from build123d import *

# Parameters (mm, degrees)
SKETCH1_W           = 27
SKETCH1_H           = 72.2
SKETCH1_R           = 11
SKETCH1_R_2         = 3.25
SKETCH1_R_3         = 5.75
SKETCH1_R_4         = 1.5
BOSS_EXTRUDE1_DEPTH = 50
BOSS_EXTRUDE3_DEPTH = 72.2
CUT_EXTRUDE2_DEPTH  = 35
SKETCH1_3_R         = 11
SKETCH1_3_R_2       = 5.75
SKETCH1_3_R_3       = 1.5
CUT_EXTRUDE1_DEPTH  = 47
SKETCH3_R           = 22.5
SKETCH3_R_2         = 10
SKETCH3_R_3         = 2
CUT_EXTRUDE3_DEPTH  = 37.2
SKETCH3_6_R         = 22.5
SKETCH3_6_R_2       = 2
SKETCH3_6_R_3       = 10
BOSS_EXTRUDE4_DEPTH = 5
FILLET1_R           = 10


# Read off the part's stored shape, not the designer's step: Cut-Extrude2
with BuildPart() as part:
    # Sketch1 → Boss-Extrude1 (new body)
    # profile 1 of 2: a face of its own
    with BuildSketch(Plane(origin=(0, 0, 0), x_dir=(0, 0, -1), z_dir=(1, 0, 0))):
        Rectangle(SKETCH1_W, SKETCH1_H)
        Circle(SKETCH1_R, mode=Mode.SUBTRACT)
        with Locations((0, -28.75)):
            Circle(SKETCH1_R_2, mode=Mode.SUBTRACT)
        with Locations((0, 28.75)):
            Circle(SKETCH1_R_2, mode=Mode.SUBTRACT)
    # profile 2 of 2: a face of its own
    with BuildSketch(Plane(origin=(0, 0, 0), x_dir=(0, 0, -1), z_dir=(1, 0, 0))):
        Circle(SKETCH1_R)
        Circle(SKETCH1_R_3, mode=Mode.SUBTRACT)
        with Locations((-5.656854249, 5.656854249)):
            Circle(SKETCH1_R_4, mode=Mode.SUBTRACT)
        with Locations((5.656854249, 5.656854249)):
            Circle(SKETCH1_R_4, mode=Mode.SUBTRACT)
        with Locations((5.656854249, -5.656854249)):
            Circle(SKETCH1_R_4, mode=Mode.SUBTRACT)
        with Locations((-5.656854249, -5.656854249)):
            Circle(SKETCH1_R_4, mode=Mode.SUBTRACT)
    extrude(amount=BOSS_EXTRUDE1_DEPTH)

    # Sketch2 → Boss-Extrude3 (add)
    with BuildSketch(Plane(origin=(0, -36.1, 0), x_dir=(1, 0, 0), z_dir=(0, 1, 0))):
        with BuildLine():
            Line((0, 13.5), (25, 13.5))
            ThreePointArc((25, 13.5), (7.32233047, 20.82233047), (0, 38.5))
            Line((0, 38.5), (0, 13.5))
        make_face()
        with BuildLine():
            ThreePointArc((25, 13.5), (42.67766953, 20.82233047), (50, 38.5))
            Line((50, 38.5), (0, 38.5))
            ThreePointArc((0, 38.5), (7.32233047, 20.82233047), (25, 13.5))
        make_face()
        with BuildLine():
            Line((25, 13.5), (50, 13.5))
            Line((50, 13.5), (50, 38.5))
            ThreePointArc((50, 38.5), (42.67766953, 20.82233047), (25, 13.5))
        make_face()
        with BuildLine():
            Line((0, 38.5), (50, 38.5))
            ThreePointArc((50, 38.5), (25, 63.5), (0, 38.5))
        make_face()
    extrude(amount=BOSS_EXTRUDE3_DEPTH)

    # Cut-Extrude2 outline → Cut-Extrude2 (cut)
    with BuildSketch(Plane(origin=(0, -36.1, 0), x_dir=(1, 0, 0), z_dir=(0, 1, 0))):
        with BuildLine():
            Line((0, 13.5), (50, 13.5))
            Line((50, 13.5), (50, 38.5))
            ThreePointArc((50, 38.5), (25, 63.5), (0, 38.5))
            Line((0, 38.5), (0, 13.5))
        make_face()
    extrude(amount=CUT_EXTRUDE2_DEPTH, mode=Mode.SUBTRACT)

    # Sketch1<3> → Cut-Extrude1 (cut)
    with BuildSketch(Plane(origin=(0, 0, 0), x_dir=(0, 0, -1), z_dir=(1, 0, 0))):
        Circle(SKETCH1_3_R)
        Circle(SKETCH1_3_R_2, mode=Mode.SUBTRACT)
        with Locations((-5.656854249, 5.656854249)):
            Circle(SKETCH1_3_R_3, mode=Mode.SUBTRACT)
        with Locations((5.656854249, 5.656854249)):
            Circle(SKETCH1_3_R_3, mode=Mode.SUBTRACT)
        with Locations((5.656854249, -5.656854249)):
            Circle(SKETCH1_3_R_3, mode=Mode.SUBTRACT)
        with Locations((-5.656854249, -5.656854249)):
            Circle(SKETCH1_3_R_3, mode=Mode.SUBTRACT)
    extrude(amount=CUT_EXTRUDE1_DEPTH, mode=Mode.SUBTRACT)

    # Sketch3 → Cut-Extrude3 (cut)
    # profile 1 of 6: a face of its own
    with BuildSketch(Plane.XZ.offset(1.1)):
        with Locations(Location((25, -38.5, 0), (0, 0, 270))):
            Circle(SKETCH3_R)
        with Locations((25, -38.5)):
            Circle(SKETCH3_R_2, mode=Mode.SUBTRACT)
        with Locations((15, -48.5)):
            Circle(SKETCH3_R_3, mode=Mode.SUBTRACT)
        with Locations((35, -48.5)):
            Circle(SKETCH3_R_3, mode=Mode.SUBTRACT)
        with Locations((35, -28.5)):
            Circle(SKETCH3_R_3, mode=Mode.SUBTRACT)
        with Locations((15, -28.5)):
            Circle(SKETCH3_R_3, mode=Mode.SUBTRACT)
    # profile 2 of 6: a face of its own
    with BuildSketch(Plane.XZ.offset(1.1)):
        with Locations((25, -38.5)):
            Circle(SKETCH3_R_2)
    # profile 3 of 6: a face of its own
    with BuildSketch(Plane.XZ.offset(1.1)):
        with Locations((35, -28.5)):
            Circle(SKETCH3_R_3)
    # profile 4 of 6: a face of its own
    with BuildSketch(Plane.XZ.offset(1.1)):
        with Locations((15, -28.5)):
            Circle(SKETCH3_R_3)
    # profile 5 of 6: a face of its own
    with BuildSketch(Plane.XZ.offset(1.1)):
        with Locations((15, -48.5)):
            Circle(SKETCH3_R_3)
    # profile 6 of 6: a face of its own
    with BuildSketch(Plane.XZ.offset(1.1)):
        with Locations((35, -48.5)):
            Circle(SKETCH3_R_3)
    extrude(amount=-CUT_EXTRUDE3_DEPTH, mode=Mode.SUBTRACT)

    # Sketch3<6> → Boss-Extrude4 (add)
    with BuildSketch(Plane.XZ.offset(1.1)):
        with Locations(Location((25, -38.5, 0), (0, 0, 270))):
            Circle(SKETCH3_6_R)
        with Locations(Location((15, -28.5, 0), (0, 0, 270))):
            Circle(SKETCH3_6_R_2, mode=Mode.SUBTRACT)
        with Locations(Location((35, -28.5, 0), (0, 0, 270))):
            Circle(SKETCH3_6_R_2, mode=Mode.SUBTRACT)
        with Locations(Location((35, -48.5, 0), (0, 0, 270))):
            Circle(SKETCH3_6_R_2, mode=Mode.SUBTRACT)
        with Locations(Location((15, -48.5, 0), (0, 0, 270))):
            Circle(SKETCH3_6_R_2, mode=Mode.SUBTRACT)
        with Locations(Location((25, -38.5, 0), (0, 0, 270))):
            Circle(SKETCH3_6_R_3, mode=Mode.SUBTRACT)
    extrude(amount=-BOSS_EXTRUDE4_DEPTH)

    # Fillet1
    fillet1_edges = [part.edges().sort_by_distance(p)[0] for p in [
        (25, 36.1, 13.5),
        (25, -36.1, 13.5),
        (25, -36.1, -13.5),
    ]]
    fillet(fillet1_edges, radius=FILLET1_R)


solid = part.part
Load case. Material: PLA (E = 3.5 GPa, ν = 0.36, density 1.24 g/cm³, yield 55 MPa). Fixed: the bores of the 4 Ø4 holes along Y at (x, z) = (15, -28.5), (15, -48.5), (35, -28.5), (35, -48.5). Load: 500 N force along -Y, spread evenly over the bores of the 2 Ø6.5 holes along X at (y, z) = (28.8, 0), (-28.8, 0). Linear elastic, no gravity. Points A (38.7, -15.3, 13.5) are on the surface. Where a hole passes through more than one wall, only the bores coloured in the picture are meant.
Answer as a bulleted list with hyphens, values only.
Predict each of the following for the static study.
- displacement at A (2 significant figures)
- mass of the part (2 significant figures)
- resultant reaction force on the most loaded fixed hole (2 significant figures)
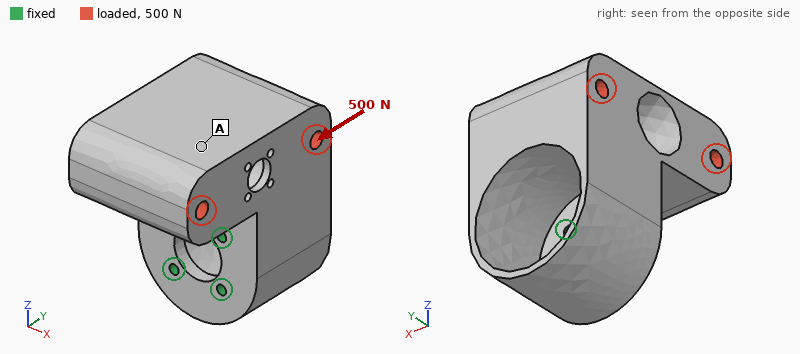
- 0.47 mm
- 130 g
- 460 N
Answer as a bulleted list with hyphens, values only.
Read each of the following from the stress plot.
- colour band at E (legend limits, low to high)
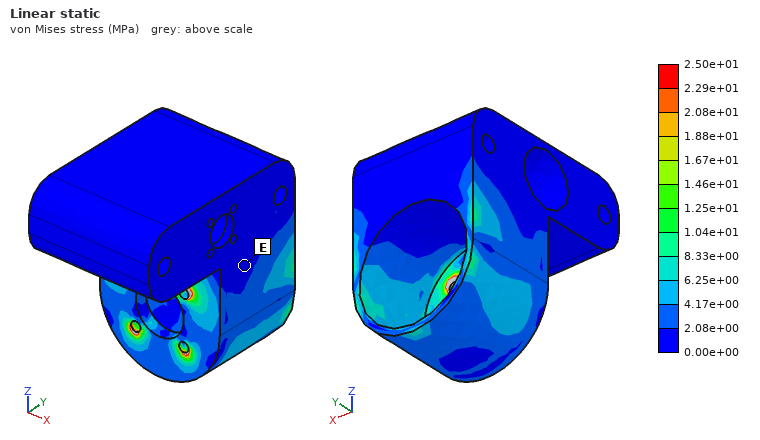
- 0.00e+00 to 2.08e+00 MPa
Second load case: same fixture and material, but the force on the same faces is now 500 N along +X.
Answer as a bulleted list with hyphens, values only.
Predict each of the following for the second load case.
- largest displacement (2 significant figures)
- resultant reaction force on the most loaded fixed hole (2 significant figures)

- 0.16 mm
- 460 N
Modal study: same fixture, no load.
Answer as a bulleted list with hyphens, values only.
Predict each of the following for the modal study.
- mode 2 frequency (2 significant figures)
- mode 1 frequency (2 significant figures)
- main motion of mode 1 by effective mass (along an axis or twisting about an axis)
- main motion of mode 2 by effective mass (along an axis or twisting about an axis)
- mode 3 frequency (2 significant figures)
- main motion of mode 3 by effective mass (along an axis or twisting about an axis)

- 790 Hz
- 520 Hz
- along Y
- twisting about Z
- 1200 Hz
- along X
